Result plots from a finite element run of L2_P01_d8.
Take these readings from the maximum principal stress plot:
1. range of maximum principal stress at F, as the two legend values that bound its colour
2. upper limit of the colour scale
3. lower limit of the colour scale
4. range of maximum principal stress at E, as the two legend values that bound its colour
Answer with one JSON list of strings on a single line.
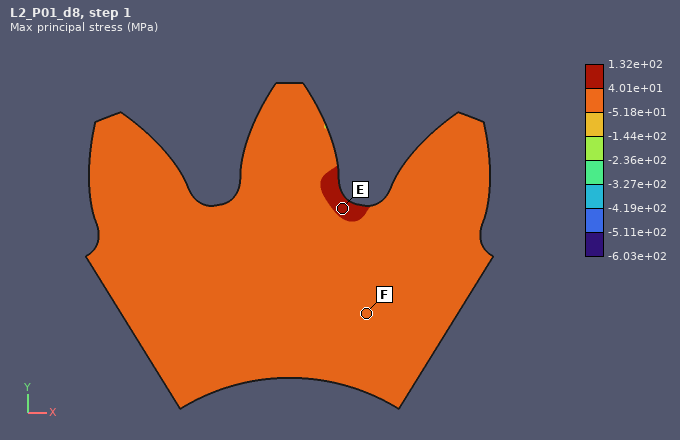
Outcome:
["-5.18e+01 to 4.01e+01 MPa", "1.32e+02 MPa", "-6.03e+02 MPa", "4.01e+01 to 1.32e+02 MPa"]
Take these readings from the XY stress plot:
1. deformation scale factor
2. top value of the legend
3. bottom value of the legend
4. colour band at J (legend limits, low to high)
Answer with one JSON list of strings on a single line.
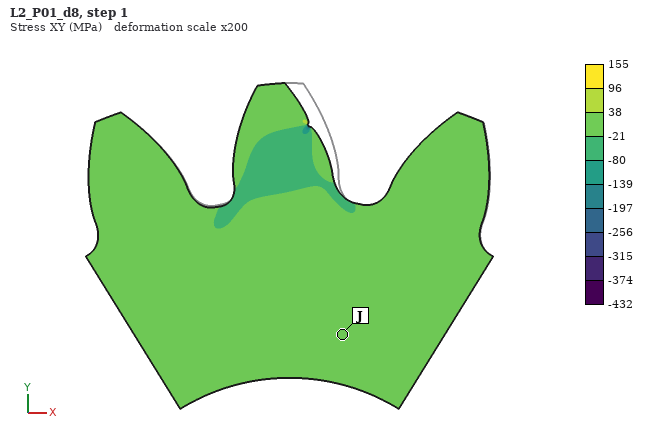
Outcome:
["200", "155 MPa", "-432 MPa", "-21 to 38 MPa"]
